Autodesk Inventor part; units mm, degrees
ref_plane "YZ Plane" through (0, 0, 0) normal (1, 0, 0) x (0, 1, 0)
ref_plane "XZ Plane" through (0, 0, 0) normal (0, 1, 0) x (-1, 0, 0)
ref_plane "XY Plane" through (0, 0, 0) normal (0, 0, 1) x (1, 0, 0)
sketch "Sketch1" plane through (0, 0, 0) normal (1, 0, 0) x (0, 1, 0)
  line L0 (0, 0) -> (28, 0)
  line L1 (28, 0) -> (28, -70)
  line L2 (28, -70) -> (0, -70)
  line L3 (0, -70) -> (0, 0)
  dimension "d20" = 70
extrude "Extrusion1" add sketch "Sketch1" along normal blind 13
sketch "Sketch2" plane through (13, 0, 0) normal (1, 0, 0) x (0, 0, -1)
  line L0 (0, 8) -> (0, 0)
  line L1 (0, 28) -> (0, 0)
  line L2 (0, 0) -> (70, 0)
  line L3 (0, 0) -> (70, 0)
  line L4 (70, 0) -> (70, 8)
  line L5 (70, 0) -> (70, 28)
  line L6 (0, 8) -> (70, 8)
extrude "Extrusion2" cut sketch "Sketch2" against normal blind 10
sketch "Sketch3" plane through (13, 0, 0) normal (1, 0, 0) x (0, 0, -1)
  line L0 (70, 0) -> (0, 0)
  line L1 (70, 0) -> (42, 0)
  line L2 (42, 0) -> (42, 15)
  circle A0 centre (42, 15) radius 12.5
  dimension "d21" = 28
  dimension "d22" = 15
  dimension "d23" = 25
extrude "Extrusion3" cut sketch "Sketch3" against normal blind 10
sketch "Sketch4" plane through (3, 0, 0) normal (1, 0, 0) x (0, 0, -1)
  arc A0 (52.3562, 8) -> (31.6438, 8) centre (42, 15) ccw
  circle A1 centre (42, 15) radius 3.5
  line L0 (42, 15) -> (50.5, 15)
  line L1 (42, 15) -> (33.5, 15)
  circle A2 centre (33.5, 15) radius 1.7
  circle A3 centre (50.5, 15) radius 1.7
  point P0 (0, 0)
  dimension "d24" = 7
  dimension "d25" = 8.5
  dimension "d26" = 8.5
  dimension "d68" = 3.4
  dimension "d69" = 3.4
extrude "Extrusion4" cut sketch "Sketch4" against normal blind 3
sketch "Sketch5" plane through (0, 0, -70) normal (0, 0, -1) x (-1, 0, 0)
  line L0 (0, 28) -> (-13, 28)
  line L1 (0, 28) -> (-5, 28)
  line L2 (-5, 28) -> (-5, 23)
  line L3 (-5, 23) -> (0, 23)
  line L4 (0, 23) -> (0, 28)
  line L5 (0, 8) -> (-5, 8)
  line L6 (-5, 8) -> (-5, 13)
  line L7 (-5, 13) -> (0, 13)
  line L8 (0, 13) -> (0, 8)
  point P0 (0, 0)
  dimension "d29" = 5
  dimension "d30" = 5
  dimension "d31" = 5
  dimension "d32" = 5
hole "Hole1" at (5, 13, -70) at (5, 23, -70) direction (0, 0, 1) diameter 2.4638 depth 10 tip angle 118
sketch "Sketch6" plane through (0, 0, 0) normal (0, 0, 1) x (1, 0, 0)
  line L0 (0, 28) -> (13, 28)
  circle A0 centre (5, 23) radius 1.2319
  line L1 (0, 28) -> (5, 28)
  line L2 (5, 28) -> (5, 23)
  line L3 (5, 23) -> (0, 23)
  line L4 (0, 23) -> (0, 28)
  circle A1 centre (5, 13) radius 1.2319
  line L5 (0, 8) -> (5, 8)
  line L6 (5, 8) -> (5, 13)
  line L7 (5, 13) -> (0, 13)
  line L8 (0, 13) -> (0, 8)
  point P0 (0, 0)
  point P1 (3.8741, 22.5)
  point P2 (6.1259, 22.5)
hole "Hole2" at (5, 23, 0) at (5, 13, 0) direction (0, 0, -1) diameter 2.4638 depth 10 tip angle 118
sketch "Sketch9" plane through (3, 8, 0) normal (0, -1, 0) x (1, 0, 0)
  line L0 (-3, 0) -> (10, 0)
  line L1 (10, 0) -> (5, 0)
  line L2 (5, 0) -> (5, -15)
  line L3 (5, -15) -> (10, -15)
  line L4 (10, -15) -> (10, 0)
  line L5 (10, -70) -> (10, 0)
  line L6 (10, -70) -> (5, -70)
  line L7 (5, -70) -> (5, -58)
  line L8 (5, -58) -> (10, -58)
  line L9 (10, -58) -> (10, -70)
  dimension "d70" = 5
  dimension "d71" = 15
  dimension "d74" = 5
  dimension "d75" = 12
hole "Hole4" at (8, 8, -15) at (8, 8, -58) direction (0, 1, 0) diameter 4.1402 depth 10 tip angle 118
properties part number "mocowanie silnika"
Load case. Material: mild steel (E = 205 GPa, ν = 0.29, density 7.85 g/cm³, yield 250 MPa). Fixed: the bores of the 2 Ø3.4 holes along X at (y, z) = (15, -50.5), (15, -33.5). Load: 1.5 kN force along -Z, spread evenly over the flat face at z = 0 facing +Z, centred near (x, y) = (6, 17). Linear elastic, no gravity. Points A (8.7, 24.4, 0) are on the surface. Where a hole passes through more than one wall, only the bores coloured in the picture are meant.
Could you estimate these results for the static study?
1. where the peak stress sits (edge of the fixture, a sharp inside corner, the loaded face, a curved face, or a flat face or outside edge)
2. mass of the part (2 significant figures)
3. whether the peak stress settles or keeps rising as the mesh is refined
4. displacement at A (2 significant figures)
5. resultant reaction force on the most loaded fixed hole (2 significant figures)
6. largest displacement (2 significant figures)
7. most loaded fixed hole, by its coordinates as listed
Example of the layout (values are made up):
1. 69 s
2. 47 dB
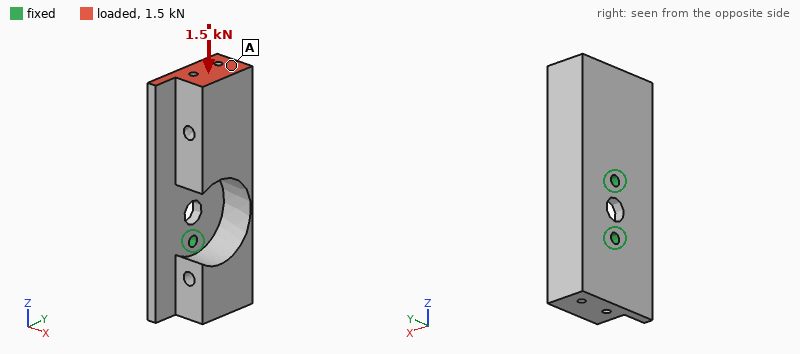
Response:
1. edge of the fixture
2. 120 g
3. keeps rising
4. 40 µm
5. 1.0 kN
6. 43 µm
7. (15, -33.5)
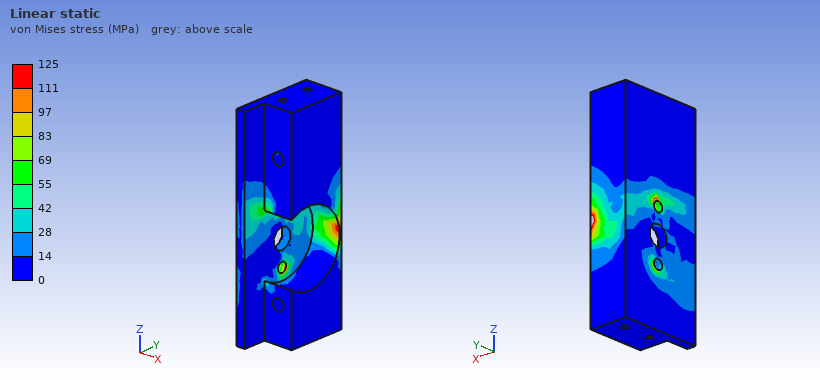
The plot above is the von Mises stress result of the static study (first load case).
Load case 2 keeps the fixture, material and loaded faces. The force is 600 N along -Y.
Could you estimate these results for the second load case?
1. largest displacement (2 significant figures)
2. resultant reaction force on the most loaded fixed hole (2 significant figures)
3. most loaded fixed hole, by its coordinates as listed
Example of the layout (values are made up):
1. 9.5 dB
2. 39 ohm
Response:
1. 29 µm
2. 1.5 kN
3. (15, -33.5)
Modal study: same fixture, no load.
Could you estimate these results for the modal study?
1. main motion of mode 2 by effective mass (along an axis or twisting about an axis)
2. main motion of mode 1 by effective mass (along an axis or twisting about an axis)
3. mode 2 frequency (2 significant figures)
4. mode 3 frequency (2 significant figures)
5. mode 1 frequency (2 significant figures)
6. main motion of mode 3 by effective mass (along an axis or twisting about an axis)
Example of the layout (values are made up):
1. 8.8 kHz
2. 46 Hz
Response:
1. along Y
2. along X
3. 4300 Hz
4. 5000 Hz
5. 2200 Hz
6. along X
